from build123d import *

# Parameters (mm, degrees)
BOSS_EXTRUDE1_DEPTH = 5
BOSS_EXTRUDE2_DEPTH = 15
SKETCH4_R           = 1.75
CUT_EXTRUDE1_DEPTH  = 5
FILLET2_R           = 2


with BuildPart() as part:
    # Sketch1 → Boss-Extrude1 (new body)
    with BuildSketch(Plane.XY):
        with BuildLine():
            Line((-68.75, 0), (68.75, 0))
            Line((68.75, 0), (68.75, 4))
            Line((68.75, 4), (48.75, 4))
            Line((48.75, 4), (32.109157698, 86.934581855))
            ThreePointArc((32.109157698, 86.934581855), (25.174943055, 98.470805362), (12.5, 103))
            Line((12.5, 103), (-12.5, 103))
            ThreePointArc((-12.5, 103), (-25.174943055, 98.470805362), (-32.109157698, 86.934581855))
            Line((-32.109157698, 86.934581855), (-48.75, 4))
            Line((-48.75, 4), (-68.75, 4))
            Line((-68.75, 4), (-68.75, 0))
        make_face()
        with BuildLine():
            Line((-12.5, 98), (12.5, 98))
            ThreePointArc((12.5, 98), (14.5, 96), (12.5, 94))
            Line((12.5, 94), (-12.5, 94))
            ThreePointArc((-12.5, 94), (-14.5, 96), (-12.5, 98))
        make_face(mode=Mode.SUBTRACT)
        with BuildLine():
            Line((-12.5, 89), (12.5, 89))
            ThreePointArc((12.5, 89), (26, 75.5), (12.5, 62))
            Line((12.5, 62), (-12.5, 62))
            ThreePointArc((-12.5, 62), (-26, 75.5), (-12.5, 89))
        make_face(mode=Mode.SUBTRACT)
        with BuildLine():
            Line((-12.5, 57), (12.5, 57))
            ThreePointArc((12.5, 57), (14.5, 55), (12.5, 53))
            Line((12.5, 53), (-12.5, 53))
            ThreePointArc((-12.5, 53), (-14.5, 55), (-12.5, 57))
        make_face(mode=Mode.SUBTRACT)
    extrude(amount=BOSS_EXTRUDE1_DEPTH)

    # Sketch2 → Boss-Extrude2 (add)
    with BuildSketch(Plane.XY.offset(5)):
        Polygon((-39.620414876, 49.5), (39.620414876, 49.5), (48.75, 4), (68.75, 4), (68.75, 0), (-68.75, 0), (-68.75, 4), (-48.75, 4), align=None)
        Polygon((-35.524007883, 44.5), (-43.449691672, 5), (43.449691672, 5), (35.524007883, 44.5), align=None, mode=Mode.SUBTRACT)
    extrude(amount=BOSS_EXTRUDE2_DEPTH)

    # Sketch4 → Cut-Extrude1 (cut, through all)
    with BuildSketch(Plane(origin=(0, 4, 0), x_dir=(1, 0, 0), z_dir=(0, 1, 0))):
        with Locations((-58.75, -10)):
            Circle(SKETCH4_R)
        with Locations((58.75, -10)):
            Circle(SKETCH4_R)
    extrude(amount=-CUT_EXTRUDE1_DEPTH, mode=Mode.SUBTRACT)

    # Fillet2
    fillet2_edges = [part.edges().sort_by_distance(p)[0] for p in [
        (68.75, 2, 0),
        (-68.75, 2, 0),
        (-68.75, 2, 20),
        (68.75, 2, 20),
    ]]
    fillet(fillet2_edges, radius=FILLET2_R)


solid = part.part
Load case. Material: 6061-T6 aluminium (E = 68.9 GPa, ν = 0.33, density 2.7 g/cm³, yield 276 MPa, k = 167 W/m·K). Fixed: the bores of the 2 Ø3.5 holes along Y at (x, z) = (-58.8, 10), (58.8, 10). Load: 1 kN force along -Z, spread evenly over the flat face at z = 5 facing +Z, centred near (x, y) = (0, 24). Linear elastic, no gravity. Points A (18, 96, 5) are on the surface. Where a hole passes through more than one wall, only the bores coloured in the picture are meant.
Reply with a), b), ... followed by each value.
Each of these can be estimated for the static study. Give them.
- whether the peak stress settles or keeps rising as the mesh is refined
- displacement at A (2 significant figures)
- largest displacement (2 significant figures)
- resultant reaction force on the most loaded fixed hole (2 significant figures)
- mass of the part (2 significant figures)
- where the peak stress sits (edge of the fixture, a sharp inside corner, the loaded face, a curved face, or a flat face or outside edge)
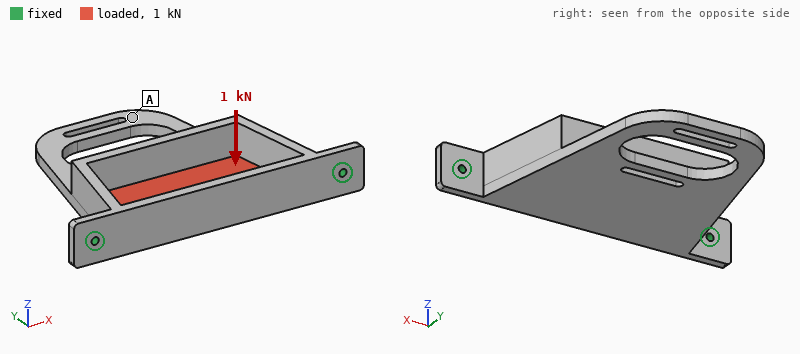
a) keeps rising
b) 1.0 mm
c) 1.1 mm
d) 530 N
e) 150 g
f) edge of the fixture
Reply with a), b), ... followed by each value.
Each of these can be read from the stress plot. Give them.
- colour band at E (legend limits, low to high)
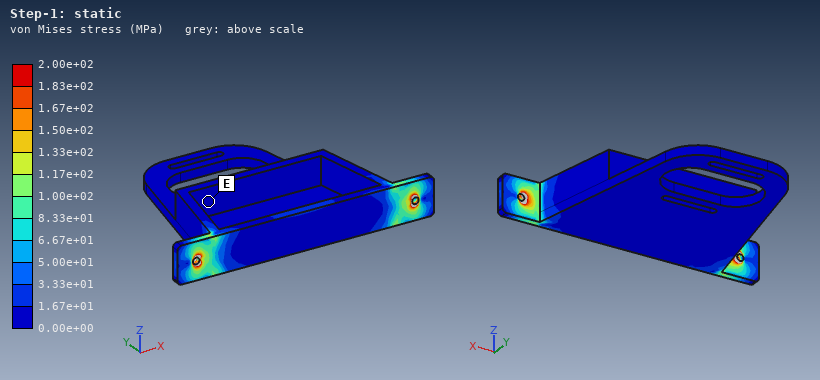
a) 0.00e+00 to 1.67e+01 MPa
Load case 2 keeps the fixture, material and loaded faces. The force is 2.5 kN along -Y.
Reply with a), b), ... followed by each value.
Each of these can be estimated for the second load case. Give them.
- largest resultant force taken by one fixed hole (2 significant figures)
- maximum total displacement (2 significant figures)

a) 1.4 kN
b) 0.61 mm
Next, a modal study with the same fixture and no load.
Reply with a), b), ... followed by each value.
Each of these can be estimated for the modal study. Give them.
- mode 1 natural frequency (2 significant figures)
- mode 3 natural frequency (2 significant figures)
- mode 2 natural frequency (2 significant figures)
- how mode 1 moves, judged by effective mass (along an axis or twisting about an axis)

a) 450 Hz
b) 1600 Hz
c) 1600 Hz
d) along Z
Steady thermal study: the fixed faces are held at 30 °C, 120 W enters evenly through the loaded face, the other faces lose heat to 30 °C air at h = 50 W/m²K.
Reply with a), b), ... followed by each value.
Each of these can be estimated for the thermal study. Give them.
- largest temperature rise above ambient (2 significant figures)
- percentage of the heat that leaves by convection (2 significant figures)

a) 66 K
b) 45 %
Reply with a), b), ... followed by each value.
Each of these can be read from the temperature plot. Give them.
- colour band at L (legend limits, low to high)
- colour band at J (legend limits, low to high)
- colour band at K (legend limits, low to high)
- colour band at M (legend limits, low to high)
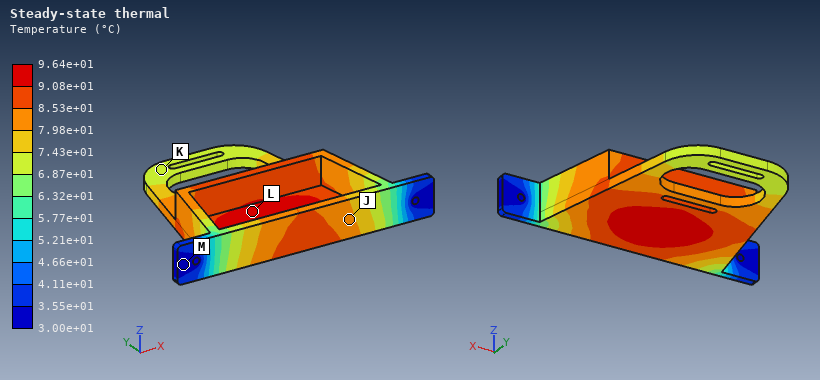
a) 9.08e+01 to 9.64e+01 °C
b) 7.98e+01 to 8.53e+01 °C
c) 6.87e+01 to 7.43e+01 °C
d) 3.00e+01 to 3.55e+01 °C
